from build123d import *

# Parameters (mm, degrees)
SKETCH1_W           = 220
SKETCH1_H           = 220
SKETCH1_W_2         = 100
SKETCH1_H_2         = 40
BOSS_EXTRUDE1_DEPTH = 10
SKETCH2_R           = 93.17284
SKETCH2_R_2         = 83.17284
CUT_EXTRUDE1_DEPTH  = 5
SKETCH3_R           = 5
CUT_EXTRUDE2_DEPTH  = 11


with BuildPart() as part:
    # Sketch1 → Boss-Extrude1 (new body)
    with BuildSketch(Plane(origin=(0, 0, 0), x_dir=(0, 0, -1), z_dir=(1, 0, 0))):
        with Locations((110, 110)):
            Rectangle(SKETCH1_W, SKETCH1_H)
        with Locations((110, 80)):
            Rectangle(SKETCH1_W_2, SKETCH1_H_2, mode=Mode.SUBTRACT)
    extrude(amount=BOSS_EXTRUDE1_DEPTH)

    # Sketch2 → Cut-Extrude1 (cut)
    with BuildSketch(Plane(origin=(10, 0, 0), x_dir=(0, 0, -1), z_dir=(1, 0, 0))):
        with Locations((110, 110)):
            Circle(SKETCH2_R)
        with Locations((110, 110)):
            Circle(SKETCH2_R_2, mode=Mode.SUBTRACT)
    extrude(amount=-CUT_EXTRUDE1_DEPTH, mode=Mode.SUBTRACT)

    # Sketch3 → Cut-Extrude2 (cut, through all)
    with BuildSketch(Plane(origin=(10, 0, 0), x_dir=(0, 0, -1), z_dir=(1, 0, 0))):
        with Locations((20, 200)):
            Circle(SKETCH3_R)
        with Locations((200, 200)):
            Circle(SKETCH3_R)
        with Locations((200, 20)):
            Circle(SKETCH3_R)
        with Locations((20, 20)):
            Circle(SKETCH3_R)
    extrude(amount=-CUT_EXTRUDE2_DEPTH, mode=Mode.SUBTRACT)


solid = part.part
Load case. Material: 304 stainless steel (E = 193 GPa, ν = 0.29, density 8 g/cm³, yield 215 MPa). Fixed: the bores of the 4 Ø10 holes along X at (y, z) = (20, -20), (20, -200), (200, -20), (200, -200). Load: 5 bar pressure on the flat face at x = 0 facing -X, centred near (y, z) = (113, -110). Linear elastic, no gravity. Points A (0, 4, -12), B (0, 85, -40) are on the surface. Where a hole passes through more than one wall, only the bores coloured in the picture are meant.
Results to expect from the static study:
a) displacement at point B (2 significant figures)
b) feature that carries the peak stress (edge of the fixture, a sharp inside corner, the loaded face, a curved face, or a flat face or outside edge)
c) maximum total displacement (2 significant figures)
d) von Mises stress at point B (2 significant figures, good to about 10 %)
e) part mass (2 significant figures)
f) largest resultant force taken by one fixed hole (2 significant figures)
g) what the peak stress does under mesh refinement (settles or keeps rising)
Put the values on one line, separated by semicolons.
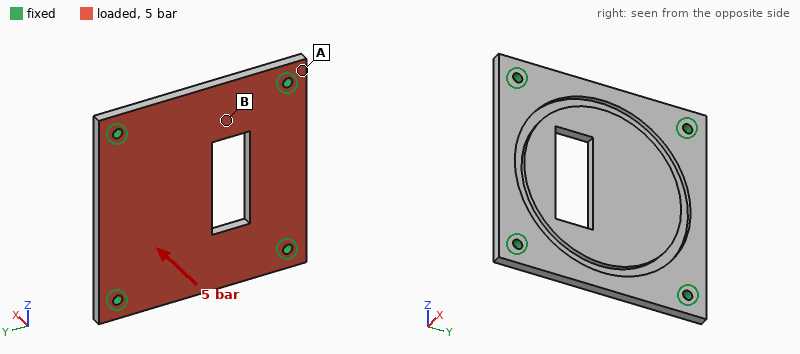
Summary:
0.16 mm; edge of the fixture; 0.30 mm; 56 MPa; 3.3 kg; 5.7 kN; keeps rising
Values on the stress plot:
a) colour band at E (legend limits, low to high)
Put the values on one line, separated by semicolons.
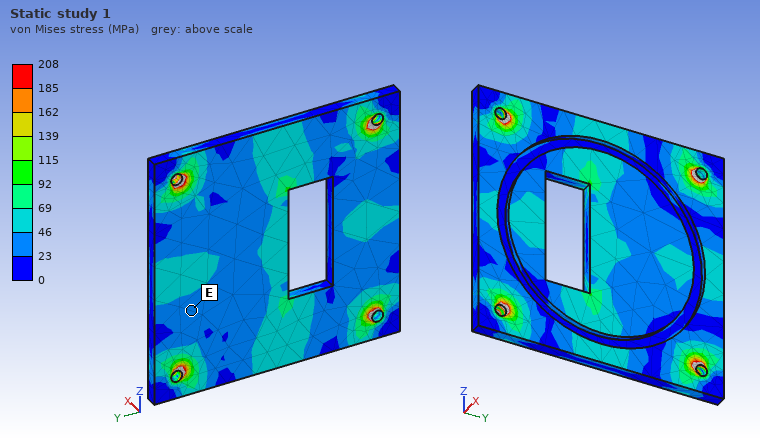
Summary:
23 to 46 MPa
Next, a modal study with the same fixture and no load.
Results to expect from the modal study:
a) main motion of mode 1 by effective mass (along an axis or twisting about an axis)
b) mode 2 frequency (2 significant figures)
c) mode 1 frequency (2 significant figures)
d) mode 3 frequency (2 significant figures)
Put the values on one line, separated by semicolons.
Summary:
along X; 1600 Hz; 1000 Hz; 1600 Hz
